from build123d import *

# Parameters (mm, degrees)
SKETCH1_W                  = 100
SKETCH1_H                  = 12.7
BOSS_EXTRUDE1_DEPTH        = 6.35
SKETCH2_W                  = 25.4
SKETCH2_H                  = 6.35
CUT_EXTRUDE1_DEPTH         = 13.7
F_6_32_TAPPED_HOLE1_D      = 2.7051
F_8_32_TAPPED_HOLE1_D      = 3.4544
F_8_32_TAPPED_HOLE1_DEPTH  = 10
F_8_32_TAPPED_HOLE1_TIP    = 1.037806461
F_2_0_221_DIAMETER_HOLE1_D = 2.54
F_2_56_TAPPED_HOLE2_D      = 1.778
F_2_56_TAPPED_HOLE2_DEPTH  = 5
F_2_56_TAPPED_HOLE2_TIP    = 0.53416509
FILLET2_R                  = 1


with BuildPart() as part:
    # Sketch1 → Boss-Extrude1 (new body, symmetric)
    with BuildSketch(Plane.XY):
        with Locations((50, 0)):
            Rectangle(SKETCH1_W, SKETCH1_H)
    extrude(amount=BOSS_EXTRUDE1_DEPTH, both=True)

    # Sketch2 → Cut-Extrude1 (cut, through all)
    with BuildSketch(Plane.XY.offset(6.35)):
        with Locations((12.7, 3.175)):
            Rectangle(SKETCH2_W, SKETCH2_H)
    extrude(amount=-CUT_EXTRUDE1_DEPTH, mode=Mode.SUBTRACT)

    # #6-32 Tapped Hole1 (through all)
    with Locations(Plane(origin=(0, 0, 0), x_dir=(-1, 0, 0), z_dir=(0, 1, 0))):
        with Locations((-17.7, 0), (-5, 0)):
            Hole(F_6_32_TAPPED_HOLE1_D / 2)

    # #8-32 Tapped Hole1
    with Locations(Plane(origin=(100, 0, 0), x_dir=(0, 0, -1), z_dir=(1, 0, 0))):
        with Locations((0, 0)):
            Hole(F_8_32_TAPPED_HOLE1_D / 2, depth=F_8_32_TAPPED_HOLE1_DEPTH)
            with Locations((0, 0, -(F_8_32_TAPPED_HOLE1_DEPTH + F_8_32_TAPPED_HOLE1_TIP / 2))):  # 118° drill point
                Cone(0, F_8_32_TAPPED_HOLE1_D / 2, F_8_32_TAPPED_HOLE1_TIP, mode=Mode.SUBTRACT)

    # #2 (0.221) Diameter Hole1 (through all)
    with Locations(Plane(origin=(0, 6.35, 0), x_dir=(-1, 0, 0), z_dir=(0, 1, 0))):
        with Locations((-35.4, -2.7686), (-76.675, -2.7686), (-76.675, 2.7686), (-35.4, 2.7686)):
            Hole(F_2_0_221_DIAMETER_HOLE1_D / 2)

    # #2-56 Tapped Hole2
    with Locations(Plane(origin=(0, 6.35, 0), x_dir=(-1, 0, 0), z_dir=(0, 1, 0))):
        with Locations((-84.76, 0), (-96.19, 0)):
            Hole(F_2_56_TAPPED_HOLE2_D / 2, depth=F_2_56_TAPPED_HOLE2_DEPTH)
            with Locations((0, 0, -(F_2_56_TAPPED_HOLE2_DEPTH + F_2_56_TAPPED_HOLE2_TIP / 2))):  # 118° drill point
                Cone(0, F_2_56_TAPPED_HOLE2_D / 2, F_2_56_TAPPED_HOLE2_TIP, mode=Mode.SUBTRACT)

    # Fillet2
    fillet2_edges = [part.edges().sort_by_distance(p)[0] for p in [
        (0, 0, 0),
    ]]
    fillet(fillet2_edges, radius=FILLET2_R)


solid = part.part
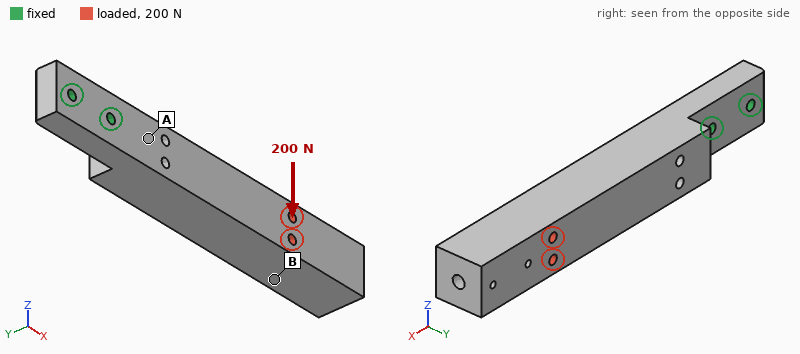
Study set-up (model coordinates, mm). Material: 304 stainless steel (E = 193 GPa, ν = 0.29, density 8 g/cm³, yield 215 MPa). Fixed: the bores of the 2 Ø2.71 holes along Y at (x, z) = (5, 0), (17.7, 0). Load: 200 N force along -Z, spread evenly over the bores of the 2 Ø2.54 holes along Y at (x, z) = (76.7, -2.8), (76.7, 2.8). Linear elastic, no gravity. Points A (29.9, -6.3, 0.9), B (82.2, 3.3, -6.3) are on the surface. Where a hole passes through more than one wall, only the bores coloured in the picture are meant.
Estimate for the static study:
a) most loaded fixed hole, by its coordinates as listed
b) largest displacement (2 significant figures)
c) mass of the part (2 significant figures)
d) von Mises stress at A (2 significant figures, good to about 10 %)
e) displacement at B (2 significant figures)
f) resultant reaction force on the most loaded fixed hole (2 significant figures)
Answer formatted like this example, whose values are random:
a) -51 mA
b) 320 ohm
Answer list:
a) (17.7, 0)
b) 0.10 mm
c) 110 g
d) 15 MPa
e) 0.078 mm
f) 840 N
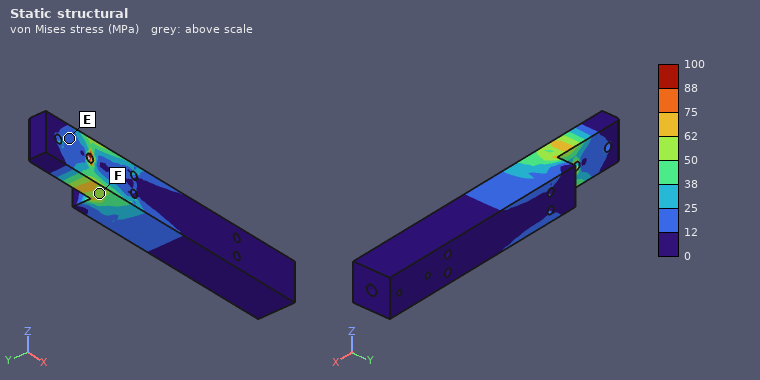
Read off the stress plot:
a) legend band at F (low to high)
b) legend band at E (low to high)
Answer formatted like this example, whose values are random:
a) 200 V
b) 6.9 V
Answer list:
a) 50 to 62 MPa
b) 12 to 25 MPa
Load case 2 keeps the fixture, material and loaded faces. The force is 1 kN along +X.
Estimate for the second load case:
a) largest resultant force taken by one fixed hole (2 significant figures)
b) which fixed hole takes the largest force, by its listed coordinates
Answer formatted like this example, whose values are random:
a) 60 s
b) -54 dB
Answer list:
a) 850 N
b) (17.7, 0)
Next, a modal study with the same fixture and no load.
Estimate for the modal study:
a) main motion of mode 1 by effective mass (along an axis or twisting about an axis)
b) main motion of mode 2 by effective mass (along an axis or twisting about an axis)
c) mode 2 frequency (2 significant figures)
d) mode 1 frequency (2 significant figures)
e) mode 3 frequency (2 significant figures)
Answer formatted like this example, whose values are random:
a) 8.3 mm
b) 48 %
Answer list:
a) along Y
b) along Z
c) 1000 Hz
d) 730 Hz
e) 5900 Hz
